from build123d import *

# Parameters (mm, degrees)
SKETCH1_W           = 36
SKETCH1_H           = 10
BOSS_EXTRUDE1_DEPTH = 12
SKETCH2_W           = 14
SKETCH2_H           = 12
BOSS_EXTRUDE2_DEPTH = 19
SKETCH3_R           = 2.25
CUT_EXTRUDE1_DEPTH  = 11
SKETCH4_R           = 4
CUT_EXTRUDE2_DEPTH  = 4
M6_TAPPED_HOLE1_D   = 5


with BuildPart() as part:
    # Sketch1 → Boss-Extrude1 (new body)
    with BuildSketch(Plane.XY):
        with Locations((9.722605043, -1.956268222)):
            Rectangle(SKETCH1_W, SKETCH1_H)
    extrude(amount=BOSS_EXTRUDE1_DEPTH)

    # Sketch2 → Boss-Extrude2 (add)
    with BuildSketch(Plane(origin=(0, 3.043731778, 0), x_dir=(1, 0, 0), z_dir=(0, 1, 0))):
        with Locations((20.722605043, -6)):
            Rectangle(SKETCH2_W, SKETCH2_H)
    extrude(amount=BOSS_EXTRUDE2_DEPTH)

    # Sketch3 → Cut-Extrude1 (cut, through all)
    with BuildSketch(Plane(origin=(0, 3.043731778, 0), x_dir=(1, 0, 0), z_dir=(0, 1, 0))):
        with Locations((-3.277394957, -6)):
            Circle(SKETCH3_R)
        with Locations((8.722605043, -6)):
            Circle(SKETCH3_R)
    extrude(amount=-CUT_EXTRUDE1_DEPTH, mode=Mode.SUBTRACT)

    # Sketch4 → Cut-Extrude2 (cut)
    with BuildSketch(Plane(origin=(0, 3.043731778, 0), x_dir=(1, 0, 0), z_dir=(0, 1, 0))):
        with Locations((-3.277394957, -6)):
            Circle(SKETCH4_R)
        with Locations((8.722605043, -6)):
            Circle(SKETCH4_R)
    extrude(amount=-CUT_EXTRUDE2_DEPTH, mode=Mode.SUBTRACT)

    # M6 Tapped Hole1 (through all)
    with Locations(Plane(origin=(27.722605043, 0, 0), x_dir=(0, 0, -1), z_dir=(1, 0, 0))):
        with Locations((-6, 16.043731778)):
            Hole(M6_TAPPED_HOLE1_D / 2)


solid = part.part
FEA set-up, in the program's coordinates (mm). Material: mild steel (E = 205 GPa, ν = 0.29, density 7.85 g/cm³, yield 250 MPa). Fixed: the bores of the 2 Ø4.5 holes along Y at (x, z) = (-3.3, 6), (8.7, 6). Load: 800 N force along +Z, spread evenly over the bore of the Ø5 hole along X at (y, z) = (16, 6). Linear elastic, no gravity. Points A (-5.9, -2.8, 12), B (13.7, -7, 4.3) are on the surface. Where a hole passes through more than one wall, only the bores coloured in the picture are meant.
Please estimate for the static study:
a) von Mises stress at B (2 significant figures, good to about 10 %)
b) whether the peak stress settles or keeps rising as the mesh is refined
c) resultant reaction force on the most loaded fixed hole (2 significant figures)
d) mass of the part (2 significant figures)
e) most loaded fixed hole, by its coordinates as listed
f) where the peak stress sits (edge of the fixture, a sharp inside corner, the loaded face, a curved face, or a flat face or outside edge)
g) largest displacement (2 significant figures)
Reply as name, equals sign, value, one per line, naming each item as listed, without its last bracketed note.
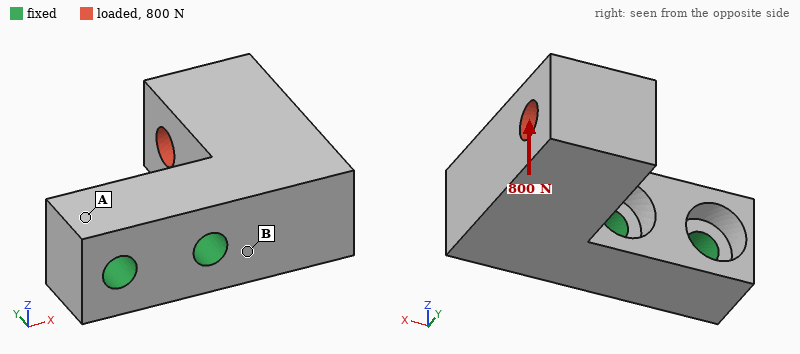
von Mises stress at B = 64 MPa
whether the peak stress settles or keeps rising as the mesh is refined = keeps rising
resultant reaction force on the most loaded fixed hole = 1.1 kN
mass of the part = 52 g
most loaded fixed hole, by its coordinates as listed = (8.7, 6)
where the peak stress sits = edge of the fixture
largest displacement = 40 µm
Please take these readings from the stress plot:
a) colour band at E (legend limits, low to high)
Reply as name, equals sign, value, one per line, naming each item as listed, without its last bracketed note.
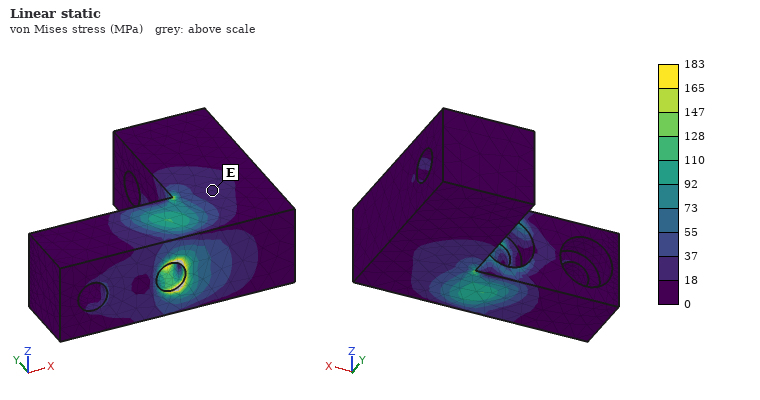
colour band at E = 18 to 37 MPa
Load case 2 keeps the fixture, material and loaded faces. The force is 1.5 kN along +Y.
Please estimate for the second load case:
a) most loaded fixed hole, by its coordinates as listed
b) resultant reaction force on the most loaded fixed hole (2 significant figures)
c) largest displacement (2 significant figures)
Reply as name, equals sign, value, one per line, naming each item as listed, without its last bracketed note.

most loaded fixed hole, by its coordinates as listed = (8.7, 6)
resultant reaction force on the most loaded fixed hole = 2.0 kN
largest displacement = 30 µm
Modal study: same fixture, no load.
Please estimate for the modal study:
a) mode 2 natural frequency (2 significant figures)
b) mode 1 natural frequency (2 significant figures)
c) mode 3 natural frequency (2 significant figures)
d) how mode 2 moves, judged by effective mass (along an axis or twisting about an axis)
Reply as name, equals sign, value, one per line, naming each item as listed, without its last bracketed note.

mode 2 natural frequency = 6200 Hz
mode 1 natural frequency = 5800 Hz
mode 3 natural frequency = 14 kHz
how mode 2 moves, judged by effective mass = along Z
